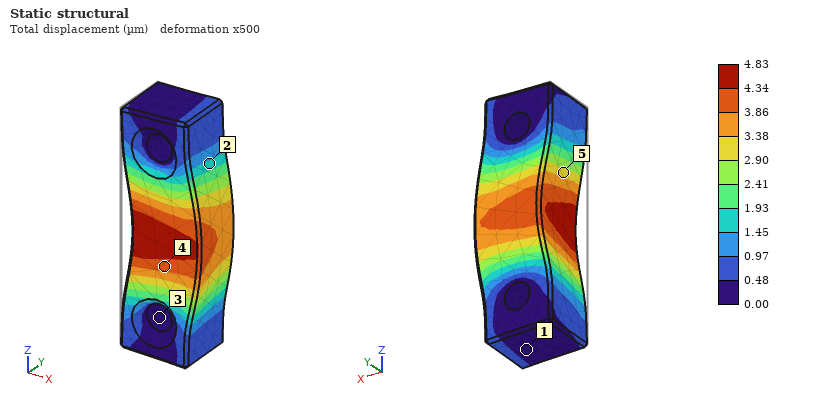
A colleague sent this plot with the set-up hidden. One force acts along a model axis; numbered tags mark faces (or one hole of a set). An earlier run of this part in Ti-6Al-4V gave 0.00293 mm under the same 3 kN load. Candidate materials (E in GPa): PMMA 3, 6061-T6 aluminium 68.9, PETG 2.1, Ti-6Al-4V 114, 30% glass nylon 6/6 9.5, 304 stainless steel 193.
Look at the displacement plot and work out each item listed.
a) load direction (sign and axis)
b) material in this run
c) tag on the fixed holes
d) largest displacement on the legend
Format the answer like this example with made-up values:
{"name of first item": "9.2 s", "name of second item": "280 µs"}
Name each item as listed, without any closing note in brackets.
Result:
{"load direction": "+X", "material in this run": "6061-T6 aluminium", "tag on the fixed holes": "3", "largest displacement on the legend": "4.83 µm"}
